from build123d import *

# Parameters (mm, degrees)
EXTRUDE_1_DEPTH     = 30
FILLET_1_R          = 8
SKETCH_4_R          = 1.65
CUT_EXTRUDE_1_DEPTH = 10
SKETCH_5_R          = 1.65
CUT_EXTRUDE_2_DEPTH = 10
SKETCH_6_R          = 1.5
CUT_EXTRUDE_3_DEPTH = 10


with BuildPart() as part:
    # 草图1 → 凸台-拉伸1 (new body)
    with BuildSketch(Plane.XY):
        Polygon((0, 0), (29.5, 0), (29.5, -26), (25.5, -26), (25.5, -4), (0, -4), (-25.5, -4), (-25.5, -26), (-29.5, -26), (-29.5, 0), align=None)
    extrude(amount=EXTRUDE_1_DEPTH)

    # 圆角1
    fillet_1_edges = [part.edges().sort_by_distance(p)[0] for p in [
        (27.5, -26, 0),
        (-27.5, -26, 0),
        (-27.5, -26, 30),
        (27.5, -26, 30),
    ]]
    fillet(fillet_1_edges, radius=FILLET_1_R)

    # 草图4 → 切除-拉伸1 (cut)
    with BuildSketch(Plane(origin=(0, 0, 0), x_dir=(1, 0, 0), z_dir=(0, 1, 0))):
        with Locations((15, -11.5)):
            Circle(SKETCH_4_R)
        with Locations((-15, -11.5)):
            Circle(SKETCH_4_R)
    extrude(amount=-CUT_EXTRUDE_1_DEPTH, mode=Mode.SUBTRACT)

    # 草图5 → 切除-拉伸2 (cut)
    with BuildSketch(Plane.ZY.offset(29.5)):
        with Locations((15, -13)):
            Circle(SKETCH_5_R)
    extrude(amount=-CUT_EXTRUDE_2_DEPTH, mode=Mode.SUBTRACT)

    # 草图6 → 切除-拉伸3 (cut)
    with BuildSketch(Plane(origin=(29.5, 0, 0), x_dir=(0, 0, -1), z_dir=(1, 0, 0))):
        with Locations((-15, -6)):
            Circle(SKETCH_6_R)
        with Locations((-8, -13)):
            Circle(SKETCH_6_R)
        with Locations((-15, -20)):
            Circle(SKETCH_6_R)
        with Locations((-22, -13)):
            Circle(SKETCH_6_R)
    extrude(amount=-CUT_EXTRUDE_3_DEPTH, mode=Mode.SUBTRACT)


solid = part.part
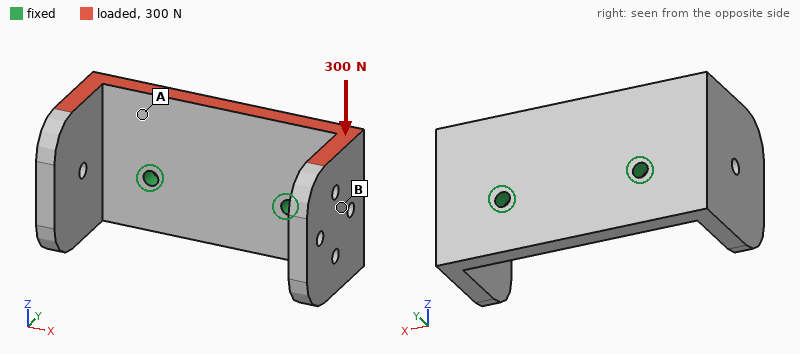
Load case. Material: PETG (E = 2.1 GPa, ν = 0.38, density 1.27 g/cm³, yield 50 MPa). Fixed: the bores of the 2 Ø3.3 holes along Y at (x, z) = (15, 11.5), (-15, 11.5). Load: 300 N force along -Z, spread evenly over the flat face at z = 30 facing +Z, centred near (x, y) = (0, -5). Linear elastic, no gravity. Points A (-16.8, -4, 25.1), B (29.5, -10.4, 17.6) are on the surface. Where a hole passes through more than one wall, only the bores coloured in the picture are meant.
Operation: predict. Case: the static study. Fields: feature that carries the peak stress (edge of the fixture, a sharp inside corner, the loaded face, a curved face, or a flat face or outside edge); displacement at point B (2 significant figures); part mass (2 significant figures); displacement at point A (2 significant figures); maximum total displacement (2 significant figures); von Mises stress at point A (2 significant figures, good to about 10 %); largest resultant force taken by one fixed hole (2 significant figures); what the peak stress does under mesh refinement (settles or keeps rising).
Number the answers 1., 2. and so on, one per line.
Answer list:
1. edge of the fixture
2. 0.14 mm
3. 15 g
4. 0.099 mm
5. 0.33 mm
6. 2.5 MPa
7. 150 N
8. keeps rising
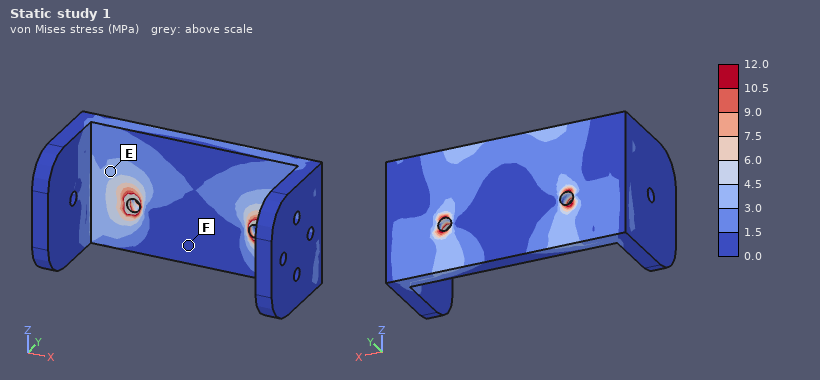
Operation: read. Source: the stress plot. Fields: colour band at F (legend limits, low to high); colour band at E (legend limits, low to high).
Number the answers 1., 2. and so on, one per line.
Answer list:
1. 0.0 to 1.5 MPa
2. 3.0 to 4.5 MPa
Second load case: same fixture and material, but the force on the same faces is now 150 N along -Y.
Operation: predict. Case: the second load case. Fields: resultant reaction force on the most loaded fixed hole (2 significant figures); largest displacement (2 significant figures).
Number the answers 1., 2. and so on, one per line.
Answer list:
1. 75 N
2. 0.81 mm
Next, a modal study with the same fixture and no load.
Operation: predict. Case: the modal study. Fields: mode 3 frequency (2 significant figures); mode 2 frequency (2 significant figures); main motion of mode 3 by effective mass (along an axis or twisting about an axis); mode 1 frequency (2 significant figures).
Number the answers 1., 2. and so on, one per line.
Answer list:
1. 970 Hz
2. 800 Hz
3. along Z
4. 780 Hz
